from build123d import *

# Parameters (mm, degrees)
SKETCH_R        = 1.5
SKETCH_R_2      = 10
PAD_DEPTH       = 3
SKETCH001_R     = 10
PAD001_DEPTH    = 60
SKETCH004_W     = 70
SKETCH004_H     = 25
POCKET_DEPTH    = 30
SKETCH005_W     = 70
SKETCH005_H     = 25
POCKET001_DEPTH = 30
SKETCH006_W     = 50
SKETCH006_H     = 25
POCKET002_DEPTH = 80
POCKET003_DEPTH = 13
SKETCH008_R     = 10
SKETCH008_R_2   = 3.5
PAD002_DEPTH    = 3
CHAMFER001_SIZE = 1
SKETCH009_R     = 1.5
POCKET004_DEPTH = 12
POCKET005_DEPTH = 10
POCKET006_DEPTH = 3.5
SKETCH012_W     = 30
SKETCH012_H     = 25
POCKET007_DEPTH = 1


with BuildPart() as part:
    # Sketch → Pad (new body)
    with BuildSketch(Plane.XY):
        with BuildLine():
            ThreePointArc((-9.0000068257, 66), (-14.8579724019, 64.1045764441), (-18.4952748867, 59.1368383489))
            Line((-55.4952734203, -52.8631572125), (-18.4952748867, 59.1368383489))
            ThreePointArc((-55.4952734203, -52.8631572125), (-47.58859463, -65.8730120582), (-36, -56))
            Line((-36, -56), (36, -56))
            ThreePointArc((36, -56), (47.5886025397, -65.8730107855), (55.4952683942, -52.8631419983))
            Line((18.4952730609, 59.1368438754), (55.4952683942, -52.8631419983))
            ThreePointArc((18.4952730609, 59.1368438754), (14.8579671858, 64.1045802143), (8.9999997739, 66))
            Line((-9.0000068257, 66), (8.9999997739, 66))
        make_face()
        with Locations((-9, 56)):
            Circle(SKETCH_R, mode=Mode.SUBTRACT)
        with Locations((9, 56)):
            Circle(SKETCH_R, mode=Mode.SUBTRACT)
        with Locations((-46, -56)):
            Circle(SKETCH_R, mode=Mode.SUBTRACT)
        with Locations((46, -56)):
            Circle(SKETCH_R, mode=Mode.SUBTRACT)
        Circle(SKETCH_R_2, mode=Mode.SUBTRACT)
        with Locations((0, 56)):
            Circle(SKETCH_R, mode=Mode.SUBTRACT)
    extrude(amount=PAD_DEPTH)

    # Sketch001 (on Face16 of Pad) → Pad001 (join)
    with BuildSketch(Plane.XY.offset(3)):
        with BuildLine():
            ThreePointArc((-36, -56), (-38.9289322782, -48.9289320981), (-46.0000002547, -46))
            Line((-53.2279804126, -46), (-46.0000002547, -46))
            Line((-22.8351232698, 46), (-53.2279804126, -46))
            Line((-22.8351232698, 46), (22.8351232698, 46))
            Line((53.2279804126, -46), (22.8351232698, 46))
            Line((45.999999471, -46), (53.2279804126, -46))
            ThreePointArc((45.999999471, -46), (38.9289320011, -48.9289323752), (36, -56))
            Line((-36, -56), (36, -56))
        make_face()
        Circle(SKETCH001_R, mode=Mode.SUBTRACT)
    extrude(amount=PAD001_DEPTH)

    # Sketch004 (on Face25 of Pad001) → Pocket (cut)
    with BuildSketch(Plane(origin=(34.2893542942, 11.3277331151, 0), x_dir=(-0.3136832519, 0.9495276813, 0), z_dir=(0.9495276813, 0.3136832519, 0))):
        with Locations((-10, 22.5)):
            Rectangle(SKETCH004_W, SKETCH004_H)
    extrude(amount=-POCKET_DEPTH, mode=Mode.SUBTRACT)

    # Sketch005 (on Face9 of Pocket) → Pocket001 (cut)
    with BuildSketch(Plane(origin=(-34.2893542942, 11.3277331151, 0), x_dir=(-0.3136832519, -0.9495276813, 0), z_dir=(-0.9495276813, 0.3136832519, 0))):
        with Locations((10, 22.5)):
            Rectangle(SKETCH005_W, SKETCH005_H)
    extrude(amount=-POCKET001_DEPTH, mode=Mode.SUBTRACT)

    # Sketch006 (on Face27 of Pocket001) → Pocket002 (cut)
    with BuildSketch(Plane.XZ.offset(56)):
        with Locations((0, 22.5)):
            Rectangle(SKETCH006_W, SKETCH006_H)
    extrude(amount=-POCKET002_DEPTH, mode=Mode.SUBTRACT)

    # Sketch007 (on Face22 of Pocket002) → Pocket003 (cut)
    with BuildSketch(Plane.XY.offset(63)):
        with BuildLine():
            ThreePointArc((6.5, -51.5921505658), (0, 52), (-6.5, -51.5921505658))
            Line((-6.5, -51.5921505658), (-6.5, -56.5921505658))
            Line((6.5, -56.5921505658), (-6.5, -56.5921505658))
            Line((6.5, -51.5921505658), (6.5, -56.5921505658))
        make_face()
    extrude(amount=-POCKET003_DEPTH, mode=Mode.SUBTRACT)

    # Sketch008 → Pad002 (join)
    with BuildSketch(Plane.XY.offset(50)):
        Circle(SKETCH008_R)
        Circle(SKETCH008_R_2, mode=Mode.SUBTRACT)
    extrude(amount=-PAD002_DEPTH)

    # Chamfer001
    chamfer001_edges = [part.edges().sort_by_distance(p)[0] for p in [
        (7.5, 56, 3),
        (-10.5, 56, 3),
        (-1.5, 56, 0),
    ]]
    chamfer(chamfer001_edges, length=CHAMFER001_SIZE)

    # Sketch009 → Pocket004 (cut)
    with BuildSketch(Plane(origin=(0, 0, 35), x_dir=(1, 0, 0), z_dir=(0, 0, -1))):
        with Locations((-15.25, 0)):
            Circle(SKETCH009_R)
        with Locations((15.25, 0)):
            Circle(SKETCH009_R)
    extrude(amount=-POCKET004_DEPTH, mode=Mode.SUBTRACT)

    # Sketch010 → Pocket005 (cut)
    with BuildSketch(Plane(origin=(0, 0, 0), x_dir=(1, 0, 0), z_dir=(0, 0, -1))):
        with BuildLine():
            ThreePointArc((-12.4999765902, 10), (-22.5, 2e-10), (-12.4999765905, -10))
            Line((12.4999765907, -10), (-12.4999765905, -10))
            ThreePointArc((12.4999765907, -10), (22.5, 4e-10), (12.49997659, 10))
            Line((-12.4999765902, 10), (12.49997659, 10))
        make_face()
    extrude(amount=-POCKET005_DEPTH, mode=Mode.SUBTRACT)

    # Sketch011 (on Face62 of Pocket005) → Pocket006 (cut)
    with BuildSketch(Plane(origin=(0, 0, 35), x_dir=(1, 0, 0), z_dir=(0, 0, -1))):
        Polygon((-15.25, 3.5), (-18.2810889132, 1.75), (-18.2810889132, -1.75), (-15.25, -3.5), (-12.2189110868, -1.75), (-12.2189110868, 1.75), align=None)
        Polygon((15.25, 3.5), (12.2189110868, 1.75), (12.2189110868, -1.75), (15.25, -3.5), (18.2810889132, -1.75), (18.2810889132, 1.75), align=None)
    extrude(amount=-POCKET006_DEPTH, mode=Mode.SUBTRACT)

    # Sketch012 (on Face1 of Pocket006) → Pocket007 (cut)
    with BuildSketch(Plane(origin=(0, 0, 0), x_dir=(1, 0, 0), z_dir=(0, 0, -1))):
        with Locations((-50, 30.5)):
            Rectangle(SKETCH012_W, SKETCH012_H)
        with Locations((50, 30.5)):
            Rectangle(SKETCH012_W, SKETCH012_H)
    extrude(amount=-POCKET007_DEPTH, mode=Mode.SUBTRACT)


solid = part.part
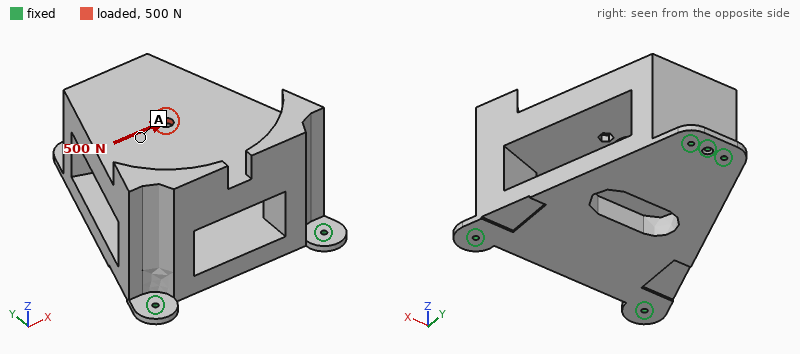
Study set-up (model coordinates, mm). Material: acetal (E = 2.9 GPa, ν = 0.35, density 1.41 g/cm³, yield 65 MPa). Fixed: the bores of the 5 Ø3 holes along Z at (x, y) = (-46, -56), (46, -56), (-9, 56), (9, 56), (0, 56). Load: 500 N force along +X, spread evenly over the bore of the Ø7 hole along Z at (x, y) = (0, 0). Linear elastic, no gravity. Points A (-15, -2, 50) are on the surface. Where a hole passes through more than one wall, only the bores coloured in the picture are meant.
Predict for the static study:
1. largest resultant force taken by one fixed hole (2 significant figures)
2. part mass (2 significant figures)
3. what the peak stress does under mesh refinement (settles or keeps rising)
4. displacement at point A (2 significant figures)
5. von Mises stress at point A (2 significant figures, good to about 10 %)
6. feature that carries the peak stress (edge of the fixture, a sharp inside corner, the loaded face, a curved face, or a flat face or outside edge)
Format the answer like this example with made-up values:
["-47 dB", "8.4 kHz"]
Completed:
["340 N", "340 g", "keeps rising", "0.39 mm", "3.0 MPa", "edge of the fixture"]
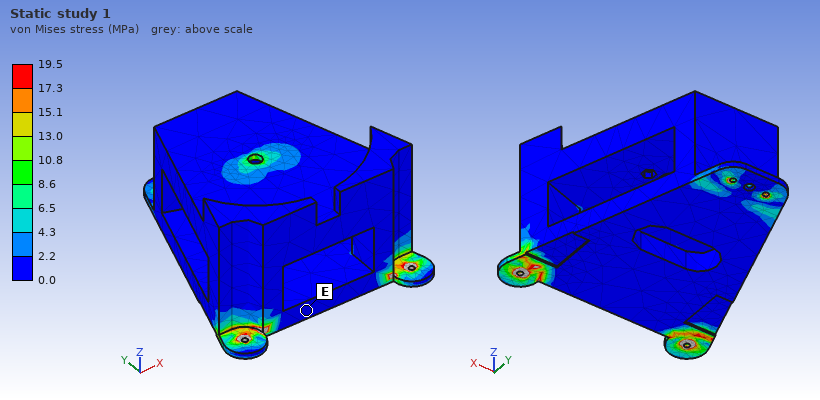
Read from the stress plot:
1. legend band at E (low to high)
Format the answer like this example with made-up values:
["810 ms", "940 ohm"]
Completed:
["0.0 to 2.2 MPa"]
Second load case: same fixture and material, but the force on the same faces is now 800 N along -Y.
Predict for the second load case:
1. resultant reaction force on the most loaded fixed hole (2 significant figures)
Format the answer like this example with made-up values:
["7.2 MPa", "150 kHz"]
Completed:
["270 N"]
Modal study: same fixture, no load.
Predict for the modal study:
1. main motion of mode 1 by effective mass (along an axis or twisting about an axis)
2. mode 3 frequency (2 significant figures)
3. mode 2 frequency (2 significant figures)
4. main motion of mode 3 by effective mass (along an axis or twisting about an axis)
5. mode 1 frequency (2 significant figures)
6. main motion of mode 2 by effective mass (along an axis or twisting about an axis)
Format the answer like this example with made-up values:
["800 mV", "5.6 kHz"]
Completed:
["along X", "540 Hz", "500 Hz", "along Y", "400 Hz", "along Z"]
